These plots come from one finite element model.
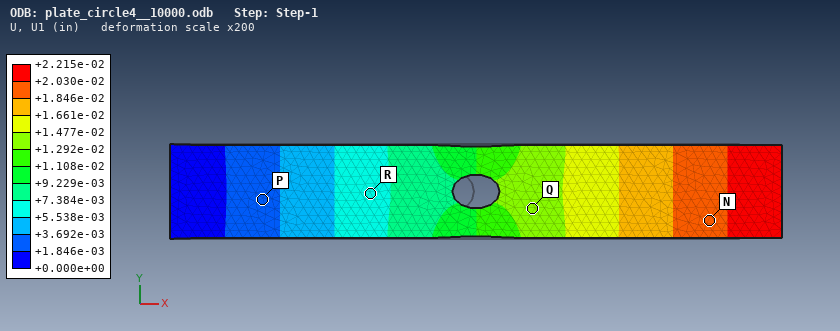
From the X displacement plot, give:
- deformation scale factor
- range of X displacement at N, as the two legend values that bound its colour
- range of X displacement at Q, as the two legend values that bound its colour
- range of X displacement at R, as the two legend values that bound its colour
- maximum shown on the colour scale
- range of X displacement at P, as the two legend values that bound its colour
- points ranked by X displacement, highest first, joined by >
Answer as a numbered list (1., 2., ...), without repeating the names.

1. 200
2. +1.846e-02 to +2.030e-02 in
3. +1.292e-02 to +1.477e-02 in
4. +5.538e-03 to +7.384e-03 in
5. +2.215e-02 in
6. +1.846e-03 to +3.692e-03 in
7. N > Q > R > P
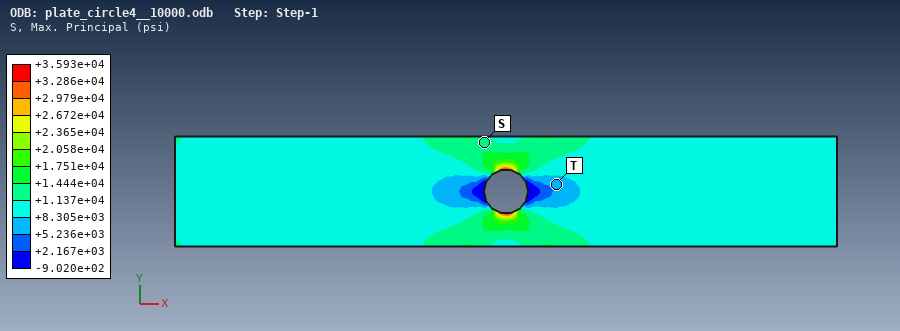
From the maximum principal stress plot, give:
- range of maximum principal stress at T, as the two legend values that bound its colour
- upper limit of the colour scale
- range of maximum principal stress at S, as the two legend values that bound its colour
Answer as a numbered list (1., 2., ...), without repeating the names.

1. +5.236e+03 to +8.305e+03 psi
2. +3.593e+04 psi
3. +1.137e+04 to +1.444e+04 psi
